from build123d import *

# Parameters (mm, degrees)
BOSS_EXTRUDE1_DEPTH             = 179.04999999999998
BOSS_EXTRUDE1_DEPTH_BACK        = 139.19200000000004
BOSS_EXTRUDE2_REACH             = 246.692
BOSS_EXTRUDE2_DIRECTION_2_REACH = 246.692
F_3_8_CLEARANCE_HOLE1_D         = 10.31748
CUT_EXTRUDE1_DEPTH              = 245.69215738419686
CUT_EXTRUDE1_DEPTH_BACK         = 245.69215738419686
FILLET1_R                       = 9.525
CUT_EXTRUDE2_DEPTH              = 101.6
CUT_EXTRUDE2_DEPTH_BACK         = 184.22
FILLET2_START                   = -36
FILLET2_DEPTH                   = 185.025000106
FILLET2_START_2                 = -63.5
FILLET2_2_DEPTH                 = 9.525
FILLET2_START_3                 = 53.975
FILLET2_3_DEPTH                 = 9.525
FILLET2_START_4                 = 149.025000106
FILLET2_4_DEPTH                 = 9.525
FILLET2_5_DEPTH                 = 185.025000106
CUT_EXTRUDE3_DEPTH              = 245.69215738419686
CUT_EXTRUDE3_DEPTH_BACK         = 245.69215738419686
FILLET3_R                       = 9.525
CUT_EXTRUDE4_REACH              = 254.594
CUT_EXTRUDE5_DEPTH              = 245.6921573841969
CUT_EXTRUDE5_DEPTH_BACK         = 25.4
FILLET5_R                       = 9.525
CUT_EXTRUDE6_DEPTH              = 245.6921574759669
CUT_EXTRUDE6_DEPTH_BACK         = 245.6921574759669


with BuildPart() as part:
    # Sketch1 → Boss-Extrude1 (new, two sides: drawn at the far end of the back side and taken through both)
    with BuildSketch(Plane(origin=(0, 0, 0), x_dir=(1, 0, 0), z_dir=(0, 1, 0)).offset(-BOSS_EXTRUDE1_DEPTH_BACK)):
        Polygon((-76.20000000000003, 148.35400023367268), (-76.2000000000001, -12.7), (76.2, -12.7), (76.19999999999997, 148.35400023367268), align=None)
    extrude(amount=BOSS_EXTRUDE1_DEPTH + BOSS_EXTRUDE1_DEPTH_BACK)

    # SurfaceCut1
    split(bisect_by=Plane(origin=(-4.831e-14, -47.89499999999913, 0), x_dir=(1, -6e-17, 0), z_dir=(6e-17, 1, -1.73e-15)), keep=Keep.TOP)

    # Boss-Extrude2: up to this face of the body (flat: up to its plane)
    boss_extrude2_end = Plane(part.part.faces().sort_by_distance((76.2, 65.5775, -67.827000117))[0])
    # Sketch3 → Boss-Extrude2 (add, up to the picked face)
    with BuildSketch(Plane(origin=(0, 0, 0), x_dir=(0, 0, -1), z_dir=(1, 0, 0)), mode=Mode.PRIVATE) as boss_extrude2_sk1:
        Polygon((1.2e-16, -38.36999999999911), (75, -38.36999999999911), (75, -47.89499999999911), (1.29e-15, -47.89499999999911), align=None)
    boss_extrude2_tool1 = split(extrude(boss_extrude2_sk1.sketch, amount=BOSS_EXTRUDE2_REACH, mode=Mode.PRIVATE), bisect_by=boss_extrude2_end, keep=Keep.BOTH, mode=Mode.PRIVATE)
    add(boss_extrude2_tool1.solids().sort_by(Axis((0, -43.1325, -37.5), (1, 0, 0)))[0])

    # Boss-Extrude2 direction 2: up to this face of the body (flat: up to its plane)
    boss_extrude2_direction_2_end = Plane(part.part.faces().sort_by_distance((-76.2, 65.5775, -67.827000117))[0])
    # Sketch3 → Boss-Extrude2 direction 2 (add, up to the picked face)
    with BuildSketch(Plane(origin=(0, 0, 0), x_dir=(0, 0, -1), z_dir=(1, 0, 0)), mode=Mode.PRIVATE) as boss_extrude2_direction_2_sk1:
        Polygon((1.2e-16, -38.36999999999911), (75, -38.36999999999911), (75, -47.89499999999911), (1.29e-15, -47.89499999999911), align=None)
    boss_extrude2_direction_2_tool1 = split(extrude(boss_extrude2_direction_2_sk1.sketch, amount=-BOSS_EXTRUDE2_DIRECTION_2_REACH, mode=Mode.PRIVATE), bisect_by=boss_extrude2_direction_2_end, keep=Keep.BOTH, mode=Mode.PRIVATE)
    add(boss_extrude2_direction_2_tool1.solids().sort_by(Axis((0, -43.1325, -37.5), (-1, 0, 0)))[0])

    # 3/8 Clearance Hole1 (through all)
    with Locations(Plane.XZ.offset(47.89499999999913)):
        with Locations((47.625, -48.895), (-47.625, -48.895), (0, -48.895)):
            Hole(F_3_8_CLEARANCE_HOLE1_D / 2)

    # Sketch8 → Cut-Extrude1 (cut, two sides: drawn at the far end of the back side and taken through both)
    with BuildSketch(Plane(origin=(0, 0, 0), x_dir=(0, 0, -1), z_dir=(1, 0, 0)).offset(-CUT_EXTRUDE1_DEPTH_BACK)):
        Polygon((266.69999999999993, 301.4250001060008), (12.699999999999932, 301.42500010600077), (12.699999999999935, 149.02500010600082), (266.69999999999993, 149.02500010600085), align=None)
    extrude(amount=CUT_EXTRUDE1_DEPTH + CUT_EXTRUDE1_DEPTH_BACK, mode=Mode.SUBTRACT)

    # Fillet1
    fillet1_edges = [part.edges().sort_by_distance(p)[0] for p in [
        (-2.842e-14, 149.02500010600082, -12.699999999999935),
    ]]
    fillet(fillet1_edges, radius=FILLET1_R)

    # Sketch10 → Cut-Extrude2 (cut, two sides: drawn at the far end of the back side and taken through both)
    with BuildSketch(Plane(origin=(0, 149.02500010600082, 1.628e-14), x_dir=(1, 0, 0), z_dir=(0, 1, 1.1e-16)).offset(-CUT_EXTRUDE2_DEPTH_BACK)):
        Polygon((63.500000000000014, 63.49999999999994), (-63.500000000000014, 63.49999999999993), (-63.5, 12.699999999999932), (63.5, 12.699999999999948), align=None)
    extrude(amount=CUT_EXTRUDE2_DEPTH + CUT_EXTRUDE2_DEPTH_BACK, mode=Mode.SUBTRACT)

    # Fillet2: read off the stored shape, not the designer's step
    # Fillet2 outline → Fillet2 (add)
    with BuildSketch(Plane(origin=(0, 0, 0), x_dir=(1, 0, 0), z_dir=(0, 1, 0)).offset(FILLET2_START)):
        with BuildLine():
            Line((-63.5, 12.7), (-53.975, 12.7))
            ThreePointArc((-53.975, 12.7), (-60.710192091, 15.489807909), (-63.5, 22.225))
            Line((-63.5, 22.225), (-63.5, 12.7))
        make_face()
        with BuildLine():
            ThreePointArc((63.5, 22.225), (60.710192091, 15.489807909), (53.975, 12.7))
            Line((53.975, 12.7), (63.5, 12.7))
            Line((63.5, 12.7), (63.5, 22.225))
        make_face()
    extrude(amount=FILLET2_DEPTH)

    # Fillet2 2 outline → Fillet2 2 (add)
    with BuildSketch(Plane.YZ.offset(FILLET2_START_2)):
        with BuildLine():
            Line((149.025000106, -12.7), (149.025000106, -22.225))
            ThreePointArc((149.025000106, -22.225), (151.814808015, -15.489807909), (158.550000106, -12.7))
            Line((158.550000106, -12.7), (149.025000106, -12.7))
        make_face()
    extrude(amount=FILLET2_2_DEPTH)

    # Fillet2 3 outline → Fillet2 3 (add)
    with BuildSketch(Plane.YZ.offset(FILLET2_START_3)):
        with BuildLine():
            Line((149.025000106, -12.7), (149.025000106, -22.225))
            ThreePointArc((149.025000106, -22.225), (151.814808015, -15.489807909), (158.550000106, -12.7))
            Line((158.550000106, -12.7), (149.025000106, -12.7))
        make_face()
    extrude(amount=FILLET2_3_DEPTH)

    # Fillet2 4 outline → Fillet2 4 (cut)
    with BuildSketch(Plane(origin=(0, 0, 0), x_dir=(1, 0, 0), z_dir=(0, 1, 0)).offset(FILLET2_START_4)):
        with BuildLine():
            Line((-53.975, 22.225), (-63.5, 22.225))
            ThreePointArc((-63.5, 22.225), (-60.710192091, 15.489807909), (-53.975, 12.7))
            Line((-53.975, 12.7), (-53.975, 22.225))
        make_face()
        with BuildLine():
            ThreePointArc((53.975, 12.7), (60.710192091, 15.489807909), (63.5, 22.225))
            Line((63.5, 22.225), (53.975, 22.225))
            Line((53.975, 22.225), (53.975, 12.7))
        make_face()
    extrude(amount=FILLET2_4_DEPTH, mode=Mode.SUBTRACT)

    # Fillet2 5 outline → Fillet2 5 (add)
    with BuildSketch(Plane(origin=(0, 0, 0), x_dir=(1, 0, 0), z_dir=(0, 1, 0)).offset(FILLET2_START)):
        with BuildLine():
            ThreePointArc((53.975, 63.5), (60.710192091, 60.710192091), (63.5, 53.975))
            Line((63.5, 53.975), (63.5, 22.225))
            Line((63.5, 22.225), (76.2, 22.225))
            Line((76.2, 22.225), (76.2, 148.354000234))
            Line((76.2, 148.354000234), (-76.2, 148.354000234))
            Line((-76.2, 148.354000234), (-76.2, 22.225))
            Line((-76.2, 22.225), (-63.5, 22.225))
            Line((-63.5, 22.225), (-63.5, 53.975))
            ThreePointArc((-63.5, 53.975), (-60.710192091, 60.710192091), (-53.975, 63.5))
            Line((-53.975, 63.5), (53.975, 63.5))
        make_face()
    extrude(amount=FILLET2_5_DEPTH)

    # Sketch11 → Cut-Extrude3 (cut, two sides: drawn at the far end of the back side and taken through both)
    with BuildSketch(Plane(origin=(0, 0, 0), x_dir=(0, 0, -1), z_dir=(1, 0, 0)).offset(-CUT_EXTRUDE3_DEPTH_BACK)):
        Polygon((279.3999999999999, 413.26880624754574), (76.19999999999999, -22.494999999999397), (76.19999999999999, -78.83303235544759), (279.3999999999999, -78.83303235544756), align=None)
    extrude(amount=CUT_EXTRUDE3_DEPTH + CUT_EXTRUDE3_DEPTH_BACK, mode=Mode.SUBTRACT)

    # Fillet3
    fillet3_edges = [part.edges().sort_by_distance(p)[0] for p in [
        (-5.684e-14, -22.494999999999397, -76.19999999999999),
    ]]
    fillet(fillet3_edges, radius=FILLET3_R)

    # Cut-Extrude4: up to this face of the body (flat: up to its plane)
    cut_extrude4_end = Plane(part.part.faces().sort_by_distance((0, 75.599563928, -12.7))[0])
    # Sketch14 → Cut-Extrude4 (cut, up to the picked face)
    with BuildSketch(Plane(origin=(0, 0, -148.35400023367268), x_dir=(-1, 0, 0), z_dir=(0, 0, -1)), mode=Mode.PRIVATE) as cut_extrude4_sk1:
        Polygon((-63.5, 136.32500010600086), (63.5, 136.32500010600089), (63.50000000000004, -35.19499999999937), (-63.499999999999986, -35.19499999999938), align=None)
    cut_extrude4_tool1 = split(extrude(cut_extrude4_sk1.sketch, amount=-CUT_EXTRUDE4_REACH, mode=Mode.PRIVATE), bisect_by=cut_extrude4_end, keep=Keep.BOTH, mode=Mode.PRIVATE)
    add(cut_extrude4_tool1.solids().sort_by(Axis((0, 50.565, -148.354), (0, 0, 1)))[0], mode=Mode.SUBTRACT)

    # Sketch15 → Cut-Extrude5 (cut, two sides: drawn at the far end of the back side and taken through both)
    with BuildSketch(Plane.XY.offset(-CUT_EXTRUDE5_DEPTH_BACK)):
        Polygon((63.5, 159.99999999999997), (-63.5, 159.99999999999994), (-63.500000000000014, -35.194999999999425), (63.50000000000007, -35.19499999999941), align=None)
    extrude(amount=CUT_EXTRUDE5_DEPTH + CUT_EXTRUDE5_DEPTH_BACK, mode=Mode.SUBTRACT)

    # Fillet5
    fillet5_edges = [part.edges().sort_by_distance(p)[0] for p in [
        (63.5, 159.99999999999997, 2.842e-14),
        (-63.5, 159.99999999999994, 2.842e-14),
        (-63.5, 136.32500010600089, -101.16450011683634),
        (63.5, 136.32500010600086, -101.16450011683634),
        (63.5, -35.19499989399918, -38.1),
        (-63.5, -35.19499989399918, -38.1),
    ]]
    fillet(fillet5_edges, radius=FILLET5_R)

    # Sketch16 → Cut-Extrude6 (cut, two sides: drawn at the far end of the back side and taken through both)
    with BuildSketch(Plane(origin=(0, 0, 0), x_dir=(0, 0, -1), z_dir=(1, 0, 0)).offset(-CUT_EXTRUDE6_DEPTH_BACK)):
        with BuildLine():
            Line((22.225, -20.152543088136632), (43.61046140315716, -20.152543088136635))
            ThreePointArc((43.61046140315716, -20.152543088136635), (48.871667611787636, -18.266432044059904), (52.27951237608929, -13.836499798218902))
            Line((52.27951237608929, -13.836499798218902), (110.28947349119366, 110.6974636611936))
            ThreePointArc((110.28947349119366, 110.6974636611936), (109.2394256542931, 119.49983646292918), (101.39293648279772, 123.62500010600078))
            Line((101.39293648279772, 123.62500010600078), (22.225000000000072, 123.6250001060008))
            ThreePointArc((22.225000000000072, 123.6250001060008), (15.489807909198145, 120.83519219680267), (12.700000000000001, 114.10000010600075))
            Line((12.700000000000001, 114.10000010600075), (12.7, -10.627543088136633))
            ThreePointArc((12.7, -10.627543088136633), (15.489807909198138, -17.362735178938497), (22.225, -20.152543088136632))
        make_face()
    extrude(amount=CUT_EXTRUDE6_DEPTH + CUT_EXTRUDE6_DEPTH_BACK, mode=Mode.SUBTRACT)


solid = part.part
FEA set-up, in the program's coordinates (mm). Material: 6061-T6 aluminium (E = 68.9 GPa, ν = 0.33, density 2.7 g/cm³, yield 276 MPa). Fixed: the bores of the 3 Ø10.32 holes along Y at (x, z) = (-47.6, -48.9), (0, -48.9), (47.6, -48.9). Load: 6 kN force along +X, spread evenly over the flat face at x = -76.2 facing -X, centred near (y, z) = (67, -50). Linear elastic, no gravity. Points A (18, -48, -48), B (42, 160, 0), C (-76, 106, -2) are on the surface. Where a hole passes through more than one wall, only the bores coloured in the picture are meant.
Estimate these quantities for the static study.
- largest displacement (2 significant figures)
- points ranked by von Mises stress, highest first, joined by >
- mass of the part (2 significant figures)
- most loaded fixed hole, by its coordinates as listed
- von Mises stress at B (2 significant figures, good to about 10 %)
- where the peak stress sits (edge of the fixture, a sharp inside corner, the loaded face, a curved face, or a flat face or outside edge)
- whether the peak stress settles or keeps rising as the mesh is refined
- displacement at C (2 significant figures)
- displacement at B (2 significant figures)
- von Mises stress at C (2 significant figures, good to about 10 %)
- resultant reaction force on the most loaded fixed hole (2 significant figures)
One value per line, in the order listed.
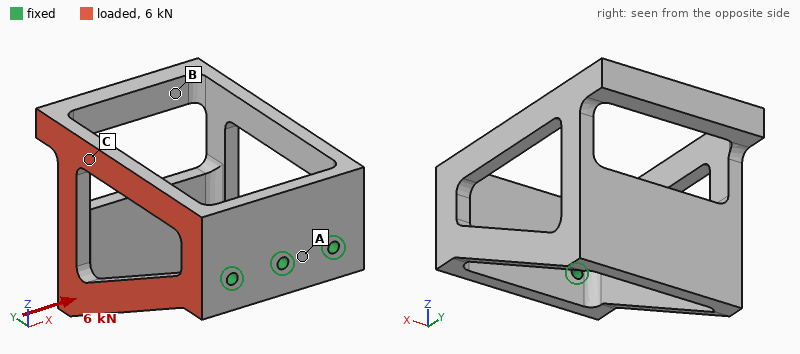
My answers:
2.1 mm
C > B > A
2.0 kg
(-47.6, -48.9)
28 MPa
edge of the fixture
keeps rising
1.8 mm
2.0 mm
68 MPa
5.2 kN
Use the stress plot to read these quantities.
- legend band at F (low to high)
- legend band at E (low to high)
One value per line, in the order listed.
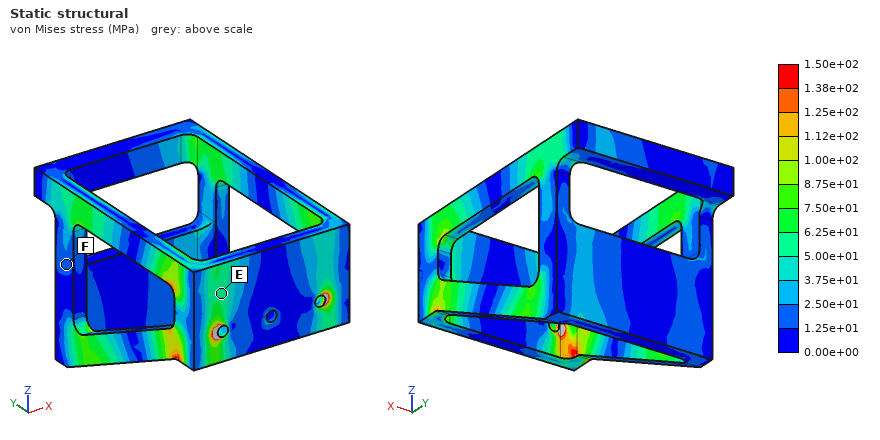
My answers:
1.25e+01 to 2.50e+01 MPa
5.00e+01 to 6.25e+01 MPa
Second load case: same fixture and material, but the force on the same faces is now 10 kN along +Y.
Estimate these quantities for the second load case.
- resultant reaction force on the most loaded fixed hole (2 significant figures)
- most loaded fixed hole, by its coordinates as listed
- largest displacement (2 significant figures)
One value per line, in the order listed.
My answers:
12 kN
(-47.6, -48.9)
0.63 mm
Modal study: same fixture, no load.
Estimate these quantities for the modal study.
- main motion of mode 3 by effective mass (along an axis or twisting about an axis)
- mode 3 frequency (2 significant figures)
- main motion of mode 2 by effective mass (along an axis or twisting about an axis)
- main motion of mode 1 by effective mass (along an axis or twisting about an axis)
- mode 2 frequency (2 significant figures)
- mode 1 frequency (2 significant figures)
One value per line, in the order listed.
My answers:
twisting about Y
390 Hz
along Z
along X
220 Hz
200 Hz
